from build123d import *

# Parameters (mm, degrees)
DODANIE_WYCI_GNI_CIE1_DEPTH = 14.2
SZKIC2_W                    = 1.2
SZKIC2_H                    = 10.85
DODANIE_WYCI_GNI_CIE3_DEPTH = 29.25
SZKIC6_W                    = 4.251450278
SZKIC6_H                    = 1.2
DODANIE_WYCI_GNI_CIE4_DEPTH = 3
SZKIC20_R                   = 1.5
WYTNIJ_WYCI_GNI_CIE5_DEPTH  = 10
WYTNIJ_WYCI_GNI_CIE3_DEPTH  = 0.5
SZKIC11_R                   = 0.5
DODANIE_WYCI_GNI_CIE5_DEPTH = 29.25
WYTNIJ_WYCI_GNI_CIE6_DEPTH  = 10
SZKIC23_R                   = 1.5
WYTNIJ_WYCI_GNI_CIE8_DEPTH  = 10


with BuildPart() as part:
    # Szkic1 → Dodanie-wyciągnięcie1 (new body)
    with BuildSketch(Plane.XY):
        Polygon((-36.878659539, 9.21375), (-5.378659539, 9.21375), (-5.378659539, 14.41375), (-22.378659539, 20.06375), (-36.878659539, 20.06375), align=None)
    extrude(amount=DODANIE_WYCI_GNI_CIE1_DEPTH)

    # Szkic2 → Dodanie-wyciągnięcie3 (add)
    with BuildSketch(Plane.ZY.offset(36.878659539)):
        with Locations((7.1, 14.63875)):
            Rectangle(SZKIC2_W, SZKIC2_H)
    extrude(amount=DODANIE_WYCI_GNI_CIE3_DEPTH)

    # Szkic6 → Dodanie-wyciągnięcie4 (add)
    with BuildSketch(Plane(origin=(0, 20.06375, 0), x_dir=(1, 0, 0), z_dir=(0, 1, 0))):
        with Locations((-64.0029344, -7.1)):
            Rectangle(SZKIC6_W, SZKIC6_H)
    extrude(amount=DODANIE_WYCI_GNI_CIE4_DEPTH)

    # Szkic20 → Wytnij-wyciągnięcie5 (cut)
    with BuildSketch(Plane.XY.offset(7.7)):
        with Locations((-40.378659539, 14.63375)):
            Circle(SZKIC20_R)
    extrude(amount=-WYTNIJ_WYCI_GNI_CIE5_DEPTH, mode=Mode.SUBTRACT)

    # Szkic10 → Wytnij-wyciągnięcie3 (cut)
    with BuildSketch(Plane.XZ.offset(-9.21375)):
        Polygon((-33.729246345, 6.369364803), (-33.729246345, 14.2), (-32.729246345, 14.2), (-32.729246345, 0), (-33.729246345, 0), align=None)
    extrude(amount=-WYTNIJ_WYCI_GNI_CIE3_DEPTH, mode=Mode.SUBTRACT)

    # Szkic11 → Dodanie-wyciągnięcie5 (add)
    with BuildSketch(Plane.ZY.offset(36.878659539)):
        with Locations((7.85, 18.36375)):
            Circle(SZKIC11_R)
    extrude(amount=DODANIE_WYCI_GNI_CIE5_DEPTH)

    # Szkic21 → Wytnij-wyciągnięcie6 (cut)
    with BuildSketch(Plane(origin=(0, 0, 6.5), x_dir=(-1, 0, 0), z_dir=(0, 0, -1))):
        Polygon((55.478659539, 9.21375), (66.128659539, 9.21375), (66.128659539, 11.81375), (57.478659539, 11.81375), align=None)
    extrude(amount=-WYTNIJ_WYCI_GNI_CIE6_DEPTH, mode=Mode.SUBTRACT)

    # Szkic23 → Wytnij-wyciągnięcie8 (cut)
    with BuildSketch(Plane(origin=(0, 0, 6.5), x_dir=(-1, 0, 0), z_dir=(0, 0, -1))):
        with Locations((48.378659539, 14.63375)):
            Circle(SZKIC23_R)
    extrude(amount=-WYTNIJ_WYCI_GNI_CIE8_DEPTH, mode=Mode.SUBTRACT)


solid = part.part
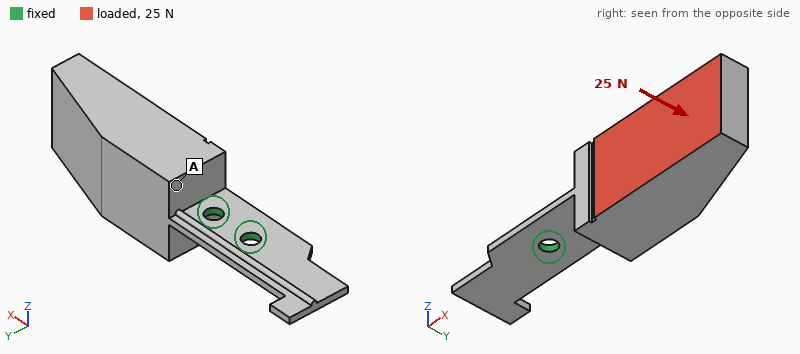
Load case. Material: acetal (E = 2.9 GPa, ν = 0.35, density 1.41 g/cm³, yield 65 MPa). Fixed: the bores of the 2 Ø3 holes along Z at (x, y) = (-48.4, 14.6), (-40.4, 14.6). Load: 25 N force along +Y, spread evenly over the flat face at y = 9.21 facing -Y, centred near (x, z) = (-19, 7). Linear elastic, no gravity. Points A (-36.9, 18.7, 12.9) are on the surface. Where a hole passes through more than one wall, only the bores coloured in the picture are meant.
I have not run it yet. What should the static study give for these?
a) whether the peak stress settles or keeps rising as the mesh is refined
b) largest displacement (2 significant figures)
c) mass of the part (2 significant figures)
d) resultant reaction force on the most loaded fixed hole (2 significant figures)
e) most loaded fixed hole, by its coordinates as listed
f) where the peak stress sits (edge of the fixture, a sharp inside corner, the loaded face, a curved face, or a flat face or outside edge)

keeps rising
0.42 mm
6.4 g
60 N
(-40.4, 14.6)
edge of the fixture
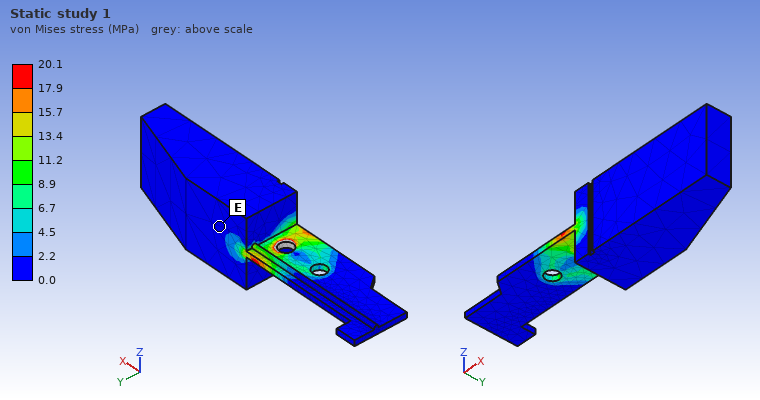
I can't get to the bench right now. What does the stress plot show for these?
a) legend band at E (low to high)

0.0 to 2.2 MPa
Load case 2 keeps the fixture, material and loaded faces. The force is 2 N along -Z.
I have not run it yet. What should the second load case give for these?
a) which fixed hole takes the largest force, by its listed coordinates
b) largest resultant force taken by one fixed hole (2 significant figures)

(-40.4, 14.6)
3.0 N
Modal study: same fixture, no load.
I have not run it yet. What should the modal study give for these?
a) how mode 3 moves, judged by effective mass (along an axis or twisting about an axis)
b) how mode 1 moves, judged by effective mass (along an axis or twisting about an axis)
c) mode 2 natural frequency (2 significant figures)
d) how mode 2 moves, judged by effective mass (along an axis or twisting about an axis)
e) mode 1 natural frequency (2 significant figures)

twisting about X
along Z
720 Hz
along Y
150 Hz
